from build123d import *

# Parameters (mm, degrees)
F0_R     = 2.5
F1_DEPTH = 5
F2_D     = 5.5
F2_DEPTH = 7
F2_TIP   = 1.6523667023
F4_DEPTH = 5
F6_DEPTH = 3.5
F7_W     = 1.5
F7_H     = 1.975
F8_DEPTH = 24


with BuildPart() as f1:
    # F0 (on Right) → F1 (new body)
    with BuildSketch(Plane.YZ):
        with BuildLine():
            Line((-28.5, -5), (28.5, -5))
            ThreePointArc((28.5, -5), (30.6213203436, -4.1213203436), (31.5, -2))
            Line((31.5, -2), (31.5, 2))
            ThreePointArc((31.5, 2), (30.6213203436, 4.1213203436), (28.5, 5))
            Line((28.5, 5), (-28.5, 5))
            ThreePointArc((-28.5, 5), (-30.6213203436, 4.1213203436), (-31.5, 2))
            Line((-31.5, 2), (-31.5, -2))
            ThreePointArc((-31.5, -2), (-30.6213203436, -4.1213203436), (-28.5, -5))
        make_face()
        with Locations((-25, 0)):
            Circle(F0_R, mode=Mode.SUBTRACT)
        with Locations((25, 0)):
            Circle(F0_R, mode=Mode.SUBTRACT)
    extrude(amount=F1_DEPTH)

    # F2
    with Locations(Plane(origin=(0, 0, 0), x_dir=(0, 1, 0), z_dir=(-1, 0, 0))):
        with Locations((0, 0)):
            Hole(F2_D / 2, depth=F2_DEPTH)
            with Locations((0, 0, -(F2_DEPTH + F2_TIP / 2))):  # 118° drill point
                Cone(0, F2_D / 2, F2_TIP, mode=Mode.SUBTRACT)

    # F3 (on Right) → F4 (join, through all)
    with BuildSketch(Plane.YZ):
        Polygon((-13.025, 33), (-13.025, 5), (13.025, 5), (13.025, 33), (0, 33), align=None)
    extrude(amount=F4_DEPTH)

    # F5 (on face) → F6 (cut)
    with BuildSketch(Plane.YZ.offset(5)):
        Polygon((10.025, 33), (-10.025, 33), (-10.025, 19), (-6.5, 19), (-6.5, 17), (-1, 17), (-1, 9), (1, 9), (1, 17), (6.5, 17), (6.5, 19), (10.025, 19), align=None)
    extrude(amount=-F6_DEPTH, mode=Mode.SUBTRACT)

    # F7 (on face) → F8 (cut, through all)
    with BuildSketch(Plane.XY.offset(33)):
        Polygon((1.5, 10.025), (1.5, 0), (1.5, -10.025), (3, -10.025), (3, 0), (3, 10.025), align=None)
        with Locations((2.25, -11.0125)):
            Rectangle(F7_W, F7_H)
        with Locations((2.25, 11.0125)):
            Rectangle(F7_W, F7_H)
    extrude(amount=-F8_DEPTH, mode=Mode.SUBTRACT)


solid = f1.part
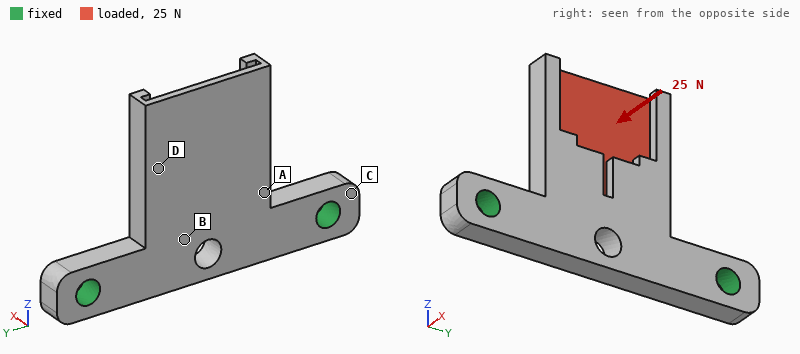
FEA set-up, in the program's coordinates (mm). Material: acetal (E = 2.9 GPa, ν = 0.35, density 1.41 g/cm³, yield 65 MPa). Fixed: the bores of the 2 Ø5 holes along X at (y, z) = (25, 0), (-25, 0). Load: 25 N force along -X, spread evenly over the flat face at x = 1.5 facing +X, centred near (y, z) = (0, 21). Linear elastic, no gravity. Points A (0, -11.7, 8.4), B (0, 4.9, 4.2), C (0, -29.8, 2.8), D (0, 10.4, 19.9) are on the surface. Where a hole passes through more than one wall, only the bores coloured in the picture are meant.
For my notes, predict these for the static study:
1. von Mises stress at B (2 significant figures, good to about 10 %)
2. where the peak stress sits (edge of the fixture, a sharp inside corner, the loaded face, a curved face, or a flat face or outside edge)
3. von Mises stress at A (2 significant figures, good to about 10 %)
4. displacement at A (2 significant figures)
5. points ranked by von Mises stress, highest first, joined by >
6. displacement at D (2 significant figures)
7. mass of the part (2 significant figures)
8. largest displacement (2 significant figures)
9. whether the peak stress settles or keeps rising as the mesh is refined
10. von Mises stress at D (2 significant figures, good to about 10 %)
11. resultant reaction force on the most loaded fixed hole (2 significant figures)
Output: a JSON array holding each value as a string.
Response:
["3.5 MPa", "a sharp inside corner", "5.2 MPa", "0.12 mm", "A > B > D > C", "0.37 mm", "7.0 g", "0.83 mm", "keeps rising", "2.0 MPa", "13 N"]
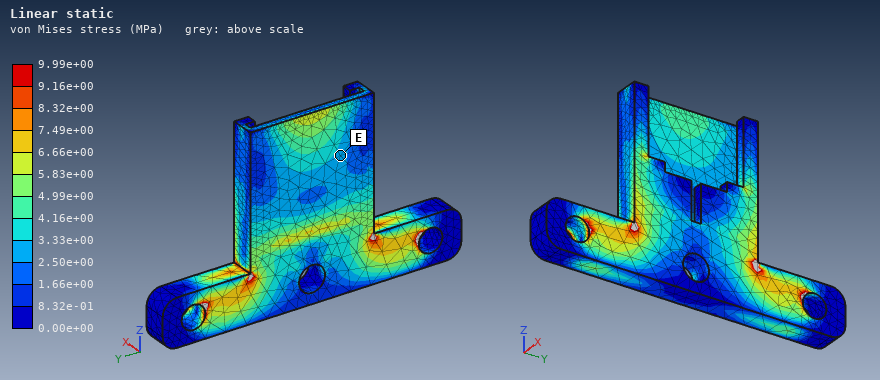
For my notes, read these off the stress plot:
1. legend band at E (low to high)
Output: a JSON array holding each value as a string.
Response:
["2.50e+00 to 3.33e+00 MPa"]
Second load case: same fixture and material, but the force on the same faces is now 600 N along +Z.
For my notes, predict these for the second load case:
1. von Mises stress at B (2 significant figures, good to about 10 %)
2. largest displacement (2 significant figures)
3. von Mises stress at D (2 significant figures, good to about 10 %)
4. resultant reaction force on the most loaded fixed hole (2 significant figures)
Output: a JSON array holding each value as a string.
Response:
["7.3 MPa", "0.62 mm", "5.3 MPa", "330 N"]
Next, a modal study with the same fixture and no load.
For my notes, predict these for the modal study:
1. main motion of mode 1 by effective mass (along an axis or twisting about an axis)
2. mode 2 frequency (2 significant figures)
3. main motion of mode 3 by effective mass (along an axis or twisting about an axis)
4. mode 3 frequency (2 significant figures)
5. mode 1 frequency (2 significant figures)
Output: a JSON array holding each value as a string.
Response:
["along X", "1800 Hz", "along X", "2600 Hz", "810 Hz"]
